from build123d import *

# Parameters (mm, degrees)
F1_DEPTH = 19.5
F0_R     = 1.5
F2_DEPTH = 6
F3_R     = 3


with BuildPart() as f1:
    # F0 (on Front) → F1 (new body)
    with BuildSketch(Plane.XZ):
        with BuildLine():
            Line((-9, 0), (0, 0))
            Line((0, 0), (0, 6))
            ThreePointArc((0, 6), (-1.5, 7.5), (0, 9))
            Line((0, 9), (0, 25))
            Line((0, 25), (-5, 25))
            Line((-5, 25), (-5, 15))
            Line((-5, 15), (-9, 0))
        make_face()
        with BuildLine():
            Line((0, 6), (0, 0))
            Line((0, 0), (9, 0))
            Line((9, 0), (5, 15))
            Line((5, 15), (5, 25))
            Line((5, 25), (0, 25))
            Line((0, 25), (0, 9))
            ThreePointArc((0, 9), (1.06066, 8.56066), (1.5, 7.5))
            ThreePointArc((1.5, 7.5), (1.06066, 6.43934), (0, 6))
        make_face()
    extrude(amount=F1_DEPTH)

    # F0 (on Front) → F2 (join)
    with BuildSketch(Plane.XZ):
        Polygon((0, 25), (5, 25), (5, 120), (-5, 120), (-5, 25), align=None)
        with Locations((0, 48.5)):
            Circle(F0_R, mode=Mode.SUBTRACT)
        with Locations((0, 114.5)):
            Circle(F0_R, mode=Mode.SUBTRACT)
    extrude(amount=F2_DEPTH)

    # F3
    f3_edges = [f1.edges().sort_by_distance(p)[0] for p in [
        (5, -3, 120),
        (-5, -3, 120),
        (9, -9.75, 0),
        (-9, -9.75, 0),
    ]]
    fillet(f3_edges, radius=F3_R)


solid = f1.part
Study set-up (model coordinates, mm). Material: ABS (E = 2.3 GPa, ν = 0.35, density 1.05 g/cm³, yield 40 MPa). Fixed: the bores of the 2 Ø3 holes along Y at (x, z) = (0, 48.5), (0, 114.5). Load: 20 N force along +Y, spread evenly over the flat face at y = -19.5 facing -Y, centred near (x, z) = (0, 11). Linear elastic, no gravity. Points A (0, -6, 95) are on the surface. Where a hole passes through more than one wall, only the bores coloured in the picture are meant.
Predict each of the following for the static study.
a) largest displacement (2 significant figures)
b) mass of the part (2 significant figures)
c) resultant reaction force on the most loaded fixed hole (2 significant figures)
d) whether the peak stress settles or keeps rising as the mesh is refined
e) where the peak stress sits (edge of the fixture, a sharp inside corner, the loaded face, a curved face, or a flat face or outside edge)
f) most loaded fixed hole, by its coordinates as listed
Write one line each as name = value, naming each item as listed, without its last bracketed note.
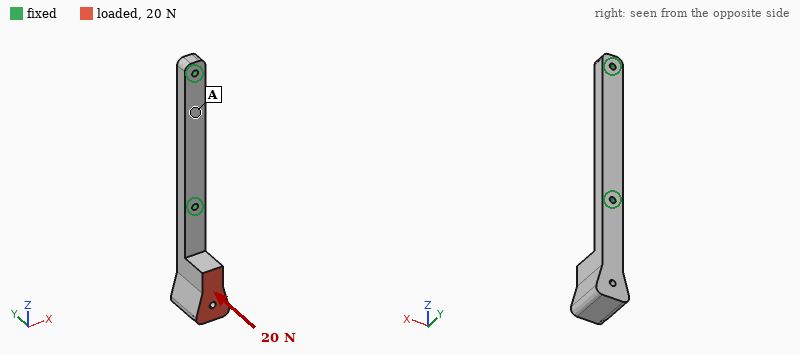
largest displacement = 1.3 mm
mass of the part = 12 g
resultant reaction force on the most loaded fixed hole = 21 N
whether the peak stress settles or keeps rising as the mesh is refined = keeps rising
where the peak stress sits = edge of the fixture
most loaded fixed hole, by its coordinates as listed = (0, 48.5)
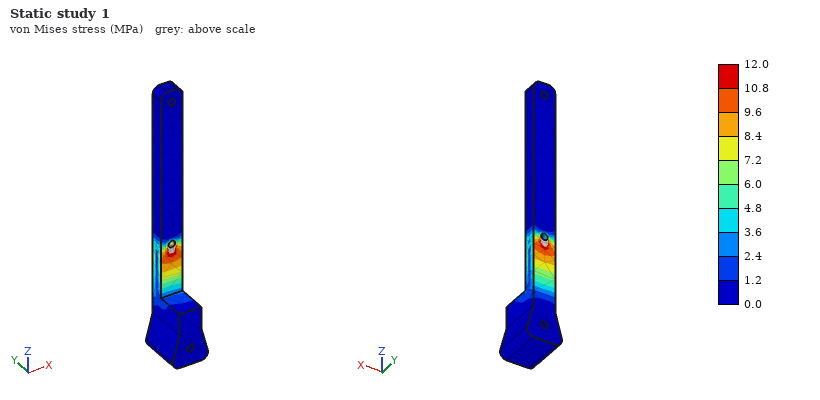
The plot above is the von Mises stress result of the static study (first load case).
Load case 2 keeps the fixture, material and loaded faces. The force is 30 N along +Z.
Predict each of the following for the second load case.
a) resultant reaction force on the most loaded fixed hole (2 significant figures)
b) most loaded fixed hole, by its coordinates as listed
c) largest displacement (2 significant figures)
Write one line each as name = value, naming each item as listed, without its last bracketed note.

resultant reaction force on the most loaded fixed hole = 29 N
most loaded fixed hole, by its coordinates as listed = (0, 48.5)
largest displacement = 1.2 mm
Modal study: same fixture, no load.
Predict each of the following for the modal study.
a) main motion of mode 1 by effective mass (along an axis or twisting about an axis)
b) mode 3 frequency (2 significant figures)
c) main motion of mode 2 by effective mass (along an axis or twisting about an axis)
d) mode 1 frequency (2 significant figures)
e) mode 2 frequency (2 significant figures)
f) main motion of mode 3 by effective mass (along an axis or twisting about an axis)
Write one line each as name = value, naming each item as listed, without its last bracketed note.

main motion of mode 1 by effective mass = along Y
mode 3 frequency = 1200 Hz
main motion of mode 2 by effective mass = along X
mode 1 frequency = 290 Hz
mode 2 frequency = 400 Hz
main motion of mode 3 by effective mass = twisting about Z
